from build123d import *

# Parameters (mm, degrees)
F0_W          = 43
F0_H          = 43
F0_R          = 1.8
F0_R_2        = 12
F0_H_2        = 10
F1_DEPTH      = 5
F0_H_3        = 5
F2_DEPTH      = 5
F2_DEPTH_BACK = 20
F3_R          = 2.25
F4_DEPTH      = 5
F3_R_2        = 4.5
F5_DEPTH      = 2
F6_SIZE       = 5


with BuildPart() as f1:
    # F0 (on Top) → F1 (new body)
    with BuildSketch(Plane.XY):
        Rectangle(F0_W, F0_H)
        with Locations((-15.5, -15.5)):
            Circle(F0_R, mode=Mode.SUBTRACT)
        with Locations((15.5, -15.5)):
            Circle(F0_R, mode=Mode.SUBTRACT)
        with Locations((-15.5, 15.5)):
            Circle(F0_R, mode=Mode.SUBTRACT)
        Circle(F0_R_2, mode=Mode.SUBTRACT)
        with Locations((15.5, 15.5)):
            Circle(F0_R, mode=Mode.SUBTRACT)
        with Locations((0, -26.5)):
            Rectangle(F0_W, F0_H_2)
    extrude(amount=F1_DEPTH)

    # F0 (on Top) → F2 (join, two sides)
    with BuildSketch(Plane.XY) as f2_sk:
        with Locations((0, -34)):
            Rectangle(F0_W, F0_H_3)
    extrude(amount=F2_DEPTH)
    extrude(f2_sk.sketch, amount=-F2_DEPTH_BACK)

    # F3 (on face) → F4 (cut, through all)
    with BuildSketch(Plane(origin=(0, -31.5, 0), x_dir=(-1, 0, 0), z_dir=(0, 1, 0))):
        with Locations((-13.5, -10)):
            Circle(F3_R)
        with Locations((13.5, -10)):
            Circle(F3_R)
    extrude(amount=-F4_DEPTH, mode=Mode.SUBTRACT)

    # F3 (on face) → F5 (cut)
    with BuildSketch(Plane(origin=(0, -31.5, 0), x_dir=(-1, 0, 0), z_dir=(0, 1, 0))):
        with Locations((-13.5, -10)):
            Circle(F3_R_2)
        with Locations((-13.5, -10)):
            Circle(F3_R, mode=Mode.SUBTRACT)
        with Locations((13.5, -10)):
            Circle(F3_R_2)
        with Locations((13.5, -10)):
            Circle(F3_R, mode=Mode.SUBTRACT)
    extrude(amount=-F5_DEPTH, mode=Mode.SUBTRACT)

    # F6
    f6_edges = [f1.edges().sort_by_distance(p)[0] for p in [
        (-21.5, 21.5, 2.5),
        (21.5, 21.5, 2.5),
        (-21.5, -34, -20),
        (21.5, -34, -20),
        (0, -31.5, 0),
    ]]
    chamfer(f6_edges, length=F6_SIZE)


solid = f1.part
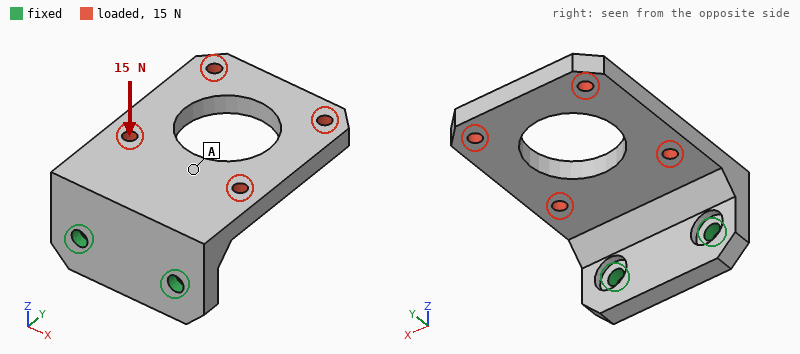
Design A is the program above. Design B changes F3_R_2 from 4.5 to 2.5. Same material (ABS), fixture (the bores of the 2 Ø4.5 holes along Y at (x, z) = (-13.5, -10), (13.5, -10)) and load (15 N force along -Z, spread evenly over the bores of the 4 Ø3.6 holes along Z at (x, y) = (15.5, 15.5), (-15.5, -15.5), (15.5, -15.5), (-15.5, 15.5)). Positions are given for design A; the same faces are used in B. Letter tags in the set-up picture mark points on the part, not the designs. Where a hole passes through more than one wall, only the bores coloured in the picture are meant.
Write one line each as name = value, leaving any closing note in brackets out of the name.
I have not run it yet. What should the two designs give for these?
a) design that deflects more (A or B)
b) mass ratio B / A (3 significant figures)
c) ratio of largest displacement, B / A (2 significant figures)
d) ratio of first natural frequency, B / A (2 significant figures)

design that deflects more = A
mass ratio B / A = 1.01
ratio of largest displacement, B / A = 0.90
ratio of first natural frequency, B / A = 1.1
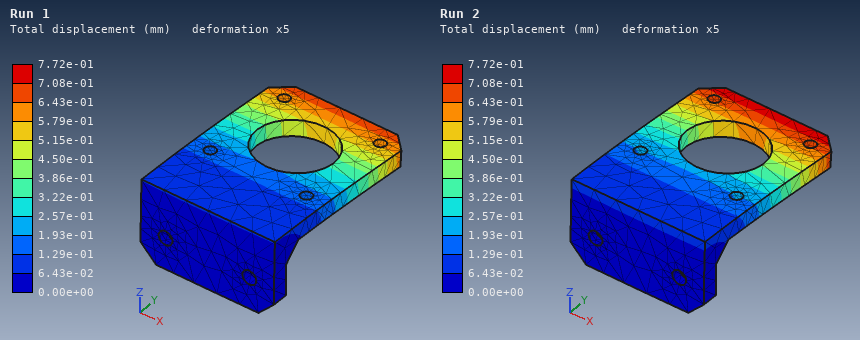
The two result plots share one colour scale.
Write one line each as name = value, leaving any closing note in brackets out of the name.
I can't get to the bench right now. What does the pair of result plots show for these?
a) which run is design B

which run is design B = Run 1
